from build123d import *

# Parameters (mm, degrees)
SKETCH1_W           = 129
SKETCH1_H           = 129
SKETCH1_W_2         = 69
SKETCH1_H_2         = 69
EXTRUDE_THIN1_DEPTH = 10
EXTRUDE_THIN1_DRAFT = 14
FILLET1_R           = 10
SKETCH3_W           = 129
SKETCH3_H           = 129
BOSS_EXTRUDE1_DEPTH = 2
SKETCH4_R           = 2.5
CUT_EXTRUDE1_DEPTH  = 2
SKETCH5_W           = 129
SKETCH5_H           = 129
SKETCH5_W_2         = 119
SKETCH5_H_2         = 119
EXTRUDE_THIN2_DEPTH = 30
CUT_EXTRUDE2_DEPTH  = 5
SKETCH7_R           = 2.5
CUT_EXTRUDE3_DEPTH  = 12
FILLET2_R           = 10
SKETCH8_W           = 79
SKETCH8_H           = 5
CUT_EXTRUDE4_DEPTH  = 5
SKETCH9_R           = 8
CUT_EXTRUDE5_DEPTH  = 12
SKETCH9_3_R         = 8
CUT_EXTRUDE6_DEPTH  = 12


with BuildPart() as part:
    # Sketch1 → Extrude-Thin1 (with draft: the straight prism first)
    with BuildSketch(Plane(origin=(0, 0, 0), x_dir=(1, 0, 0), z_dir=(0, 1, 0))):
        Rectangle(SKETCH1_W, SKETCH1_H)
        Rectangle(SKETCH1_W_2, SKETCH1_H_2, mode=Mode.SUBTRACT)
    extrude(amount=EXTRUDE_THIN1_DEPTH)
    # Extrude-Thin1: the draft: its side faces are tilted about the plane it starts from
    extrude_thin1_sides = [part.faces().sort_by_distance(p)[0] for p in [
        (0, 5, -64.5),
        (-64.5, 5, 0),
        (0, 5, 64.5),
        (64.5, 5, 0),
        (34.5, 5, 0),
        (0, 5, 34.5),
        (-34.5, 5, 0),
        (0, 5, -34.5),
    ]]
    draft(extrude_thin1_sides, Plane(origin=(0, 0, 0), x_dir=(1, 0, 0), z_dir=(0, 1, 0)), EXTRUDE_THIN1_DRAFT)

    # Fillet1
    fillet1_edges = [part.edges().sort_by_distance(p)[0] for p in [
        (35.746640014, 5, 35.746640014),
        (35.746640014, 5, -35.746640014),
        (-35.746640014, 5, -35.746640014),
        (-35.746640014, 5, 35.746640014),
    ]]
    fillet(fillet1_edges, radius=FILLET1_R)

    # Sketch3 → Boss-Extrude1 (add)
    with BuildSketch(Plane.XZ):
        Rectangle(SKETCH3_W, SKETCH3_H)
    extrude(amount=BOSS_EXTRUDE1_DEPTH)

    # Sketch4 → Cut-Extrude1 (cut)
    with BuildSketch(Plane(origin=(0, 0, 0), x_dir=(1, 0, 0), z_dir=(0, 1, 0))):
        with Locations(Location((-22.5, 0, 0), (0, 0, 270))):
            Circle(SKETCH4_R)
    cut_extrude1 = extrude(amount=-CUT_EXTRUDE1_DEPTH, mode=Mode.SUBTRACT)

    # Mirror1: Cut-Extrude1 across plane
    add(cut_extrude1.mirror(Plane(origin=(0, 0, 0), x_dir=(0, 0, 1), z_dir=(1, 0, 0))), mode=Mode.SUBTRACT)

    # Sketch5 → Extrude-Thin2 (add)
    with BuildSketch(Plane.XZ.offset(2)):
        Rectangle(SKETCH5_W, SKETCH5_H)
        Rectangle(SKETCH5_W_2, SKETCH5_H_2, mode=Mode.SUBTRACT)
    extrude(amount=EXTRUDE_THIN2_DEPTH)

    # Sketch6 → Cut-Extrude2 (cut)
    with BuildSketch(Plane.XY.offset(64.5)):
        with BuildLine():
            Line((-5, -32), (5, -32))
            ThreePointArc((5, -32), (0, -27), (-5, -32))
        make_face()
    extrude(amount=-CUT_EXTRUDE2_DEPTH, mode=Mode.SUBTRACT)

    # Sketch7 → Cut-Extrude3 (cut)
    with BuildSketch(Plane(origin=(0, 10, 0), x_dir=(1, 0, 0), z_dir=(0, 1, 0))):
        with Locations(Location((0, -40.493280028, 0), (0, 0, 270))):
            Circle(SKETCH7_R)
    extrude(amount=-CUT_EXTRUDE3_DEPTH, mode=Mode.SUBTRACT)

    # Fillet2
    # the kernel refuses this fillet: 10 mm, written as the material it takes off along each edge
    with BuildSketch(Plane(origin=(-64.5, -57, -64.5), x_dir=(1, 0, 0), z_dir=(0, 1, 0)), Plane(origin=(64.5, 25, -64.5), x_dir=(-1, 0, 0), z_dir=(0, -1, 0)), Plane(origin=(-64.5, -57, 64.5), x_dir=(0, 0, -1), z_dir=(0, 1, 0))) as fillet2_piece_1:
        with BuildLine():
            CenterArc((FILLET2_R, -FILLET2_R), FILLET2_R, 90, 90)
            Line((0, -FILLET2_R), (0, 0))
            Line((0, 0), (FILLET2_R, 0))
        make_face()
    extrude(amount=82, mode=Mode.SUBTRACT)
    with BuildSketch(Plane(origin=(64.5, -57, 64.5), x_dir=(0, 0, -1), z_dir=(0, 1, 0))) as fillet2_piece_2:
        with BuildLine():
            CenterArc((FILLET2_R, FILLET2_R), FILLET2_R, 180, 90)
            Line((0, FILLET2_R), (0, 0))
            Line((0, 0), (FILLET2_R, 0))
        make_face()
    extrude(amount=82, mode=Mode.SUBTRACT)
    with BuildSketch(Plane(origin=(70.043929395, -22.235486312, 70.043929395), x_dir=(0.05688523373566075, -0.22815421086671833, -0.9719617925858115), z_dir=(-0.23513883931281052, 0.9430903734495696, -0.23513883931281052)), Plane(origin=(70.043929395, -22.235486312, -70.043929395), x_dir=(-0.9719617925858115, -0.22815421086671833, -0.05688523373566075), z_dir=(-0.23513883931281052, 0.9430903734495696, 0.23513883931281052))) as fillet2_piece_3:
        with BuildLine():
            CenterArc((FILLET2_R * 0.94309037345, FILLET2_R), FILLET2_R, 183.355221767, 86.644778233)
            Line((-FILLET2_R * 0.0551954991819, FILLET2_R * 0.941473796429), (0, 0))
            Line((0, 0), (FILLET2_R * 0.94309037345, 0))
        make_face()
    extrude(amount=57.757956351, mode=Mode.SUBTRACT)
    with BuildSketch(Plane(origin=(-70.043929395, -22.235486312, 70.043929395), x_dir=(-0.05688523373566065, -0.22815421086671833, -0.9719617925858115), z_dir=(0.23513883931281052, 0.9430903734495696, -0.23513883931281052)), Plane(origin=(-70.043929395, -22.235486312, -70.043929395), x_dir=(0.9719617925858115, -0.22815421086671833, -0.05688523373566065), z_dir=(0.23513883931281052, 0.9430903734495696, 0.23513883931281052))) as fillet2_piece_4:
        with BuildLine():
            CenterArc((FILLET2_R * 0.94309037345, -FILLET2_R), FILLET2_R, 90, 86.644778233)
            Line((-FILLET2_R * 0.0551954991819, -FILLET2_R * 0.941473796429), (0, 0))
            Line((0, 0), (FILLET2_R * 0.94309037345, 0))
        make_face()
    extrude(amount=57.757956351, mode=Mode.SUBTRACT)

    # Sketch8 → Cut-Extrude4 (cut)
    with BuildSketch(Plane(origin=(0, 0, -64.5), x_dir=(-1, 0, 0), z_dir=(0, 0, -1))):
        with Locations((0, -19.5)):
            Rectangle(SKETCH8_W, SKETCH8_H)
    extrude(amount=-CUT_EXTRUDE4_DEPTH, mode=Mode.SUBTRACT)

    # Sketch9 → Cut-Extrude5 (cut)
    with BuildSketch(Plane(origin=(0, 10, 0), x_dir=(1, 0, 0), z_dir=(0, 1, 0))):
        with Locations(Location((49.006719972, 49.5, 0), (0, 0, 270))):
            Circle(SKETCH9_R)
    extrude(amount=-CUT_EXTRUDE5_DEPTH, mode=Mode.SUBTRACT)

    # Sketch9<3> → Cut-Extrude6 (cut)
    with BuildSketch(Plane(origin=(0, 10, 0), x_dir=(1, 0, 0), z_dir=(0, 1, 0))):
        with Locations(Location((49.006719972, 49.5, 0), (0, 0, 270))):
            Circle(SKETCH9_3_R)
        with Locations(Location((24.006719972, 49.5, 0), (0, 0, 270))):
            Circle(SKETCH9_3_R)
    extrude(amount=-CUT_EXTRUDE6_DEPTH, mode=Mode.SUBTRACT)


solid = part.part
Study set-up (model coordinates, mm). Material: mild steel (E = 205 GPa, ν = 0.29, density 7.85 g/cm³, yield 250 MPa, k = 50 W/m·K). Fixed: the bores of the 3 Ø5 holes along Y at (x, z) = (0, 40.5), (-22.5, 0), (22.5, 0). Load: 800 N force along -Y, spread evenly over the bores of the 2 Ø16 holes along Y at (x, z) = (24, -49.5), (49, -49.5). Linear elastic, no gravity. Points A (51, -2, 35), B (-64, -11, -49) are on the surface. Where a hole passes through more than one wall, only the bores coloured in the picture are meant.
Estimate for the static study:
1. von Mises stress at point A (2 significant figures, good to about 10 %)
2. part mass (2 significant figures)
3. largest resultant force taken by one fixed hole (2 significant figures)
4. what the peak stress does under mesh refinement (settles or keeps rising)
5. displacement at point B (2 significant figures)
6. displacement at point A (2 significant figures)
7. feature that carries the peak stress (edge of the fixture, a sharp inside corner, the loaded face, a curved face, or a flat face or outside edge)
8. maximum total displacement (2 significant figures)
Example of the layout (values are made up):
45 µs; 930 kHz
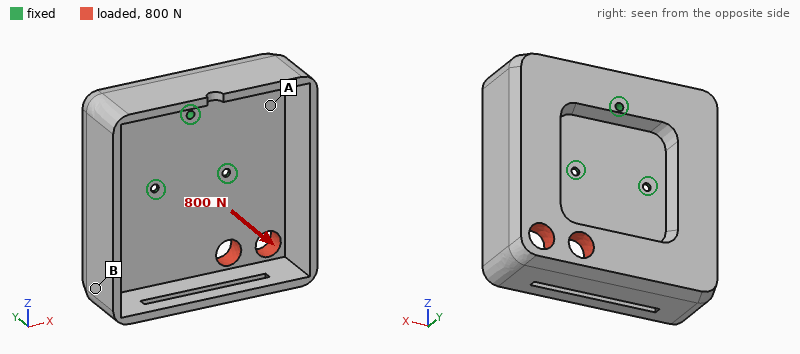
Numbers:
18 MPa; 1.6 kg; 1.3 kN; keeps rising; 0.023 mm; 0.021 mm; edge of the fixture; 0.13 mm
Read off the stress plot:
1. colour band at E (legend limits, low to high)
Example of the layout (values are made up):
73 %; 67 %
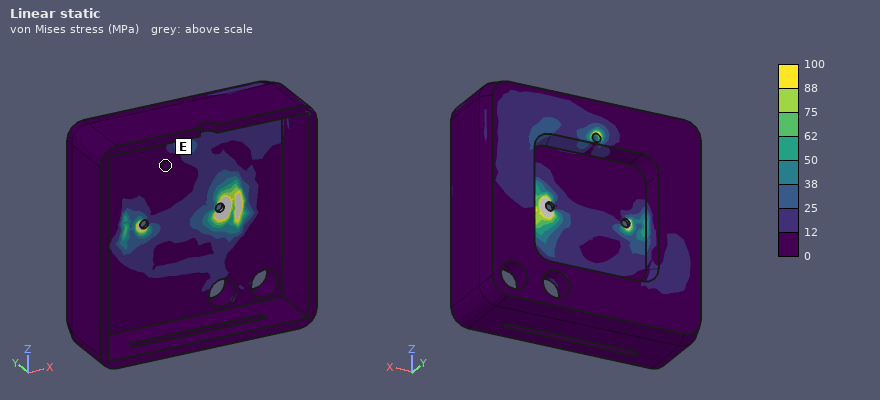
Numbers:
0 to 12 MPa
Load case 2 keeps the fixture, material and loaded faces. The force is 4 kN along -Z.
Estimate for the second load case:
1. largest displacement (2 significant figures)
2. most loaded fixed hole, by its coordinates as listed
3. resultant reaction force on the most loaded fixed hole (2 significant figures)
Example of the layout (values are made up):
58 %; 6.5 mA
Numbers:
21 µm; (22.5, 0); 3.0 kN
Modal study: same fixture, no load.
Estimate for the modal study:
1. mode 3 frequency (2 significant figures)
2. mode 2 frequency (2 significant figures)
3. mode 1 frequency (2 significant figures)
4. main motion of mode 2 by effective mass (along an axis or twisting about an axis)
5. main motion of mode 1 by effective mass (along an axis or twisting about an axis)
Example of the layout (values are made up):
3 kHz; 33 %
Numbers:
1600 Hz; 780 Hz; 660 Hz; twisting about Z; along Y
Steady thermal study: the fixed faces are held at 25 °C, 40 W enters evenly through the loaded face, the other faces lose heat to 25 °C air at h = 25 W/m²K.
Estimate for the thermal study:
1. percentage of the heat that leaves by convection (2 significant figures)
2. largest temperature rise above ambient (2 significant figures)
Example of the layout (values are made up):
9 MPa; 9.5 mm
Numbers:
69 %; 56 K
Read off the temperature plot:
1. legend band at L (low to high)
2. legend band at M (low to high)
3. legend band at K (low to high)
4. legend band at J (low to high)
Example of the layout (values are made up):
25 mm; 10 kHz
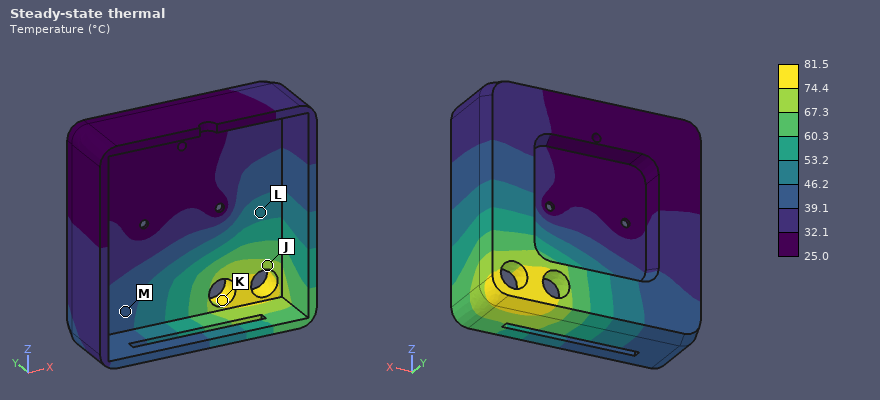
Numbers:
46.2 to 53.2 °C; 39.1 to 46.2 °C; 74.4 to 81.5 °C; 67.3 to 74.4 °C
